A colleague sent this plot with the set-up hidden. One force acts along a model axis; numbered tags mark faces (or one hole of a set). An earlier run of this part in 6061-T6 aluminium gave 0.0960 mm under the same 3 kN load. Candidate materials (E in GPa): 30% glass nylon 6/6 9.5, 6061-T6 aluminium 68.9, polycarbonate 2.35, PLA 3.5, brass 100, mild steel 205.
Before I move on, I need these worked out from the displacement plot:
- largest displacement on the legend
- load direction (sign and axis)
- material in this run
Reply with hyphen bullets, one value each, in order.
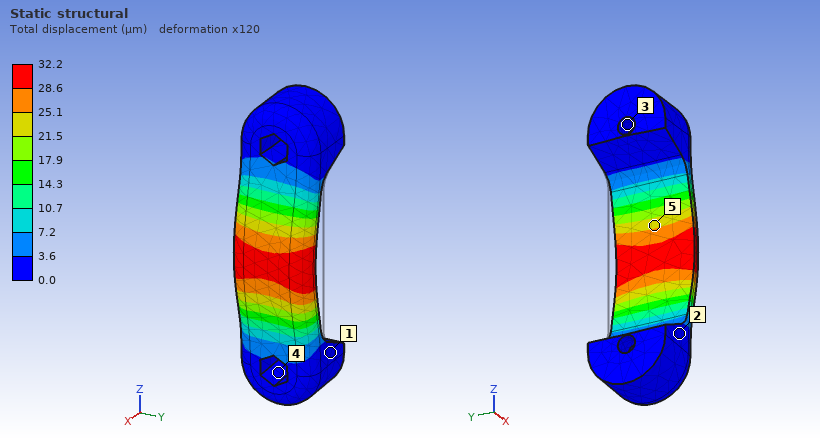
- 32.2 µm
- +X
- mild steel
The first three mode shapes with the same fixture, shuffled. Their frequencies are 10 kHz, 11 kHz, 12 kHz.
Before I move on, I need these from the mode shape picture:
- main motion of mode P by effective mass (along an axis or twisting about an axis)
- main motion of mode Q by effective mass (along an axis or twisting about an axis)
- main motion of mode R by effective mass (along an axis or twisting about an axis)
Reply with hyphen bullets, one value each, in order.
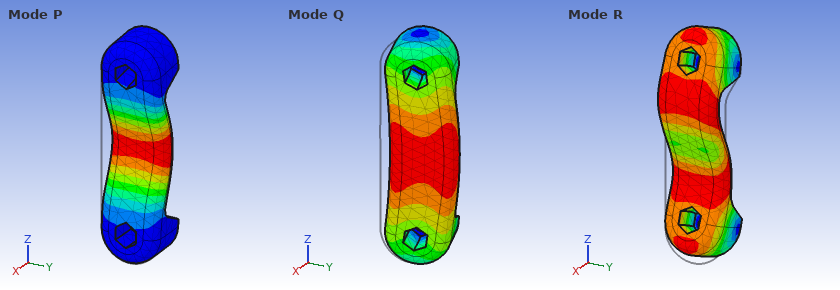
- along X
- along Y
- along Z
